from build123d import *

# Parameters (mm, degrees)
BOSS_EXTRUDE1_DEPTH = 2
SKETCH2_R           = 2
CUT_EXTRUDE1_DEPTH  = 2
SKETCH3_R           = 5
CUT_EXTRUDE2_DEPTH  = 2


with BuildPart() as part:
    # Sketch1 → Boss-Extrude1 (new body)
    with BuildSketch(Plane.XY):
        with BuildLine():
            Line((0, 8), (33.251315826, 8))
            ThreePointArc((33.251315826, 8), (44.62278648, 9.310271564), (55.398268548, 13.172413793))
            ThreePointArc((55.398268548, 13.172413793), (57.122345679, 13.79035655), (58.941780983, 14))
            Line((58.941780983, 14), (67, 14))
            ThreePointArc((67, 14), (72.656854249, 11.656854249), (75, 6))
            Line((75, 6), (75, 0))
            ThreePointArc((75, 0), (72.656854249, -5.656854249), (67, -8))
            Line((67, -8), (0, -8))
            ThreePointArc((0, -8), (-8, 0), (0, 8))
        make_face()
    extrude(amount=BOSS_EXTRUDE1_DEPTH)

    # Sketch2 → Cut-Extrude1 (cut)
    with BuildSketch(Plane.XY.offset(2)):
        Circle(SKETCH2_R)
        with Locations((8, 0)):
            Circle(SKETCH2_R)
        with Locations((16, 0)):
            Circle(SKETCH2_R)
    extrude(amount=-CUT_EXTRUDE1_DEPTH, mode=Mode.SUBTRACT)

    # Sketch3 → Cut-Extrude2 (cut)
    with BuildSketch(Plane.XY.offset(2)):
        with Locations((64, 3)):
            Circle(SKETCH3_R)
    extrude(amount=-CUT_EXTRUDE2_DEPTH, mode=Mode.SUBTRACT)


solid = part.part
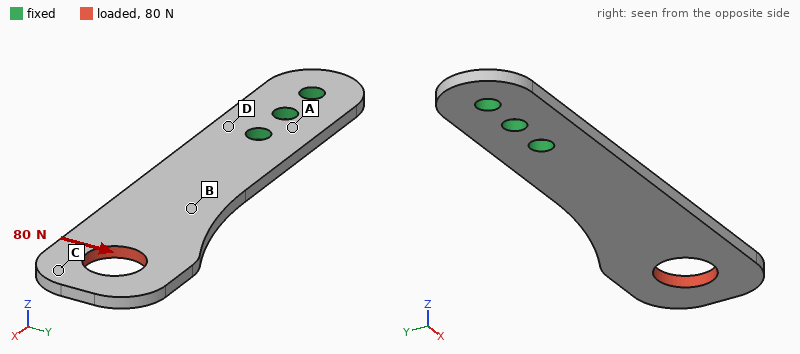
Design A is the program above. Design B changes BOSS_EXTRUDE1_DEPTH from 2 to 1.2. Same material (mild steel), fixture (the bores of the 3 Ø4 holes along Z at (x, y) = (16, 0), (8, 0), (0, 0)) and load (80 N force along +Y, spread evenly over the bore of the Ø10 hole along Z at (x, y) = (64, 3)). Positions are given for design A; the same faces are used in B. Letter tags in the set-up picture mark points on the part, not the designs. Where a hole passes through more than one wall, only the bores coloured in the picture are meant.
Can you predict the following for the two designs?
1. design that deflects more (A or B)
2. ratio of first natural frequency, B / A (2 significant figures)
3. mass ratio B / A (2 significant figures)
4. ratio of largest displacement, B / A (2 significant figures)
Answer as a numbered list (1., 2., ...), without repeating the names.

1. B
2. 0.60
3. 0.60
4. 1.7
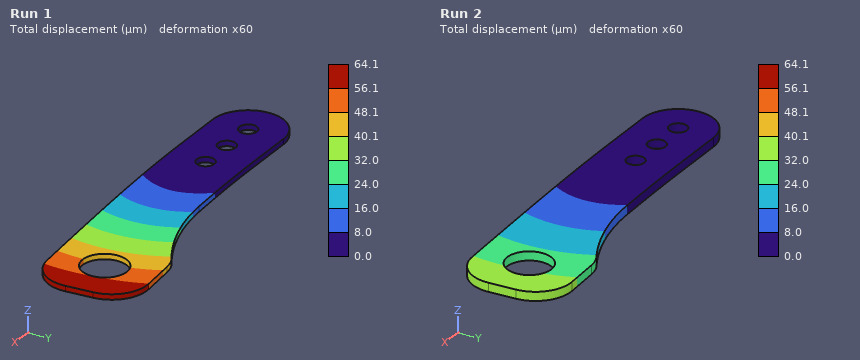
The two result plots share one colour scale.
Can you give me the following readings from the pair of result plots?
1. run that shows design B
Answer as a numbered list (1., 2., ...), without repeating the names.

1. Run 1
